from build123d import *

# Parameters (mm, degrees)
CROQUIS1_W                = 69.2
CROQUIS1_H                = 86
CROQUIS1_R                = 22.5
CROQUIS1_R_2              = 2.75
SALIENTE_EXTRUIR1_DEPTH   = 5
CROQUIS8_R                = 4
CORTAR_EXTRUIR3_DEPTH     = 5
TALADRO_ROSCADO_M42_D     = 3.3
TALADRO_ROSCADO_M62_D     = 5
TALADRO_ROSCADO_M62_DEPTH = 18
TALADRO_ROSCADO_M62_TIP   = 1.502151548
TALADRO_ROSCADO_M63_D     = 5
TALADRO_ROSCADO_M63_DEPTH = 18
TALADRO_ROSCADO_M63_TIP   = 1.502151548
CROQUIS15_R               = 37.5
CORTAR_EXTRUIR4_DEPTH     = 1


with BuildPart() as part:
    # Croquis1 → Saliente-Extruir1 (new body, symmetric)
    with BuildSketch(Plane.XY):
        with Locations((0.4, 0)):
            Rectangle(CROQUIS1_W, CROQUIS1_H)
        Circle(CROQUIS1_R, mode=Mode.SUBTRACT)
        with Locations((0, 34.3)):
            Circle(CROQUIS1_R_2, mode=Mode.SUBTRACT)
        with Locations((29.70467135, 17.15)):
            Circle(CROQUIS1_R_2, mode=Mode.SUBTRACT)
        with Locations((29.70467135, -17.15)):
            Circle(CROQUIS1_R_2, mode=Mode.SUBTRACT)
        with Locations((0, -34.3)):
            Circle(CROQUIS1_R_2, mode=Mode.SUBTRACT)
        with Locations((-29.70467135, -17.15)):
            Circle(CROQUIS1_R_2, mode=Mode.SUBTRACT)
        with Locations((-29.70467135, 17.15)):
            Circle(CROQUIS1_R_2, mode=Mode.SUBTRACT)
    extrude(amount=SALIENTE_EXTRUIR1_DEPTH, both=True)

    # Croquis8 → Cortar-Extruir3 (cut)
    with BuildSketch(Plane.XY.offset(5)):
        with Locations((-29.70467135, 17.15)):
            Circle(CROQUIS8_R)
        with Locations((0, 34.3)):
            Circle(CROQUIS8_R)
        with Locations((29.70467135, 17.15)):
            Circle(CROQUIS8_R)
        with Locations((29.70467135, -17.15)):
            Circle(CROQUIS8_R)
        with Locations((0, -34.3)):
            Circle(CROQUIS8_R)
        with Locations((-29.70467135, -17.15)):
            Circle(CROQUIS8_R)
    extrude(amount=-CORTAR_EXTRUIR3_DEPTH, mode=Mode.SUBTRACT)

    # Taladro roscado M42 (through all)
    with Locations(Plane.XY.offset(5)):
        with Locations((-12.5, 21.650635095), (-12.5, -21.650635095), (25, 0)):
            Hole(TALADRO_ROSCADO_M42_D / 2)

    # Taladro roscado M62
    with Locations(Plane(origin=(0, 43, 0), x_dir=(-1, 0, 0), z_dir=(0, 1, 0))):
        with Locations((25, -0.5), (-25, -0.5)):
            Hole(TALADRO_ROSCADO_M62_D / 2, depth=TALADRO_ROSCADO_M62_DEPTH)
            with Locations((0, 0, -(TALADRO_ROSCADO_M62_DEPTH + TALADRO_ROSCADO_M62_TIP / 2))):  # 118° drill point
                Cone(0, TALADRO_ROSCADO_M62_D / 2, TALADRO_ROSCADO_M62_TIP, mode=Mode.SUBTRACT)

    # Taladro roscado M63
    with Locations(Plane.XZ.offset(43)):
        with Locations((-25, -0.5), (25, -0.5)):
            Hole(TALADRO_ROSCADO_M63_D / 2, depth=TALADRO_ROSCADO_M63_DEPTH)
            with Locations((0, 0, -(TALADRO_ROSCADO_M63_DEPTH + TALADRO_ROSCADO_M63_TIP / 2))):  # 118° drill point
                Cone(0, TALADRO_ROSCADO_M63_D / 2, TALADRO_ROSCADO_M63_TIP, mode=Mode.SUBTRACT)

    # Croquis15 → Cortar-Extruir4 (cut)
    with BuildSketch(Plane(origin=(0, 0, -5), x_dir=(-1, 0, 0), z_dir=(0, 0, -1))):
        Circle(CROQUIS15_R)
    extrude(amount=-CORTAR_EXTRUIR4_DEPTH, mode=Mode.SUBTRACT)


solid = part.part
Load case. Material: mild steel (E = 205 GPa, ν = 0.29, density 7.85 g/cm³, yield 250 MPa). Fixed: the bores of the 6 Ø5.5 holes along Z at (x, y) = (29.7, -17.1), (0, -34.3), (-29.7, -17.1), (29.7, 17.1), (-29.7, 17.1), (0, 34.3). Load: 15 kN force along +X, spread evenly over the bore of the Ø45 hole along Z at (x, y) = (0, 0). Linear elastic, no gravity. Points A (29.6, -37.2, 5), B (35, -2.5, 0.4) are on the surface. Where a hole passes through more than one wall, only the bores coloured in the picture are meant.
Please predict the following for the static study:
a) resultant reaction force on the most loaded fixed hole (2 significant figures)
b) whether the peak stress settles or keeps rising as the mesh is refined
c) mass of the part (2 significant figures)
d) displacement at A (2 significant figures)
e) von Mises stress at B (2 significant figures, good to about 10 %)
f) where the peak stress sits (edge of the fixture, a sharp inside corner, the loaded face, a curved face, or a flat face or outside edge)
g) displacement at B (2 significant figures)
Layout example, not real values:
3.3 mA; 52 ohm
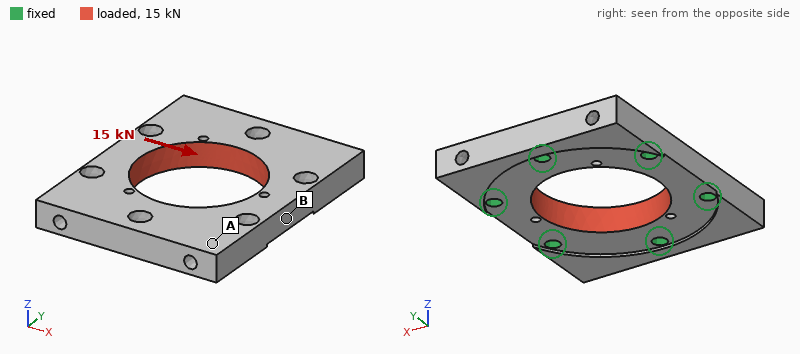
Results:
2.7 kN; keeps rising; 290 g; 2.4 µm; 21 MPa; edge of the fixture; 3.1 µm
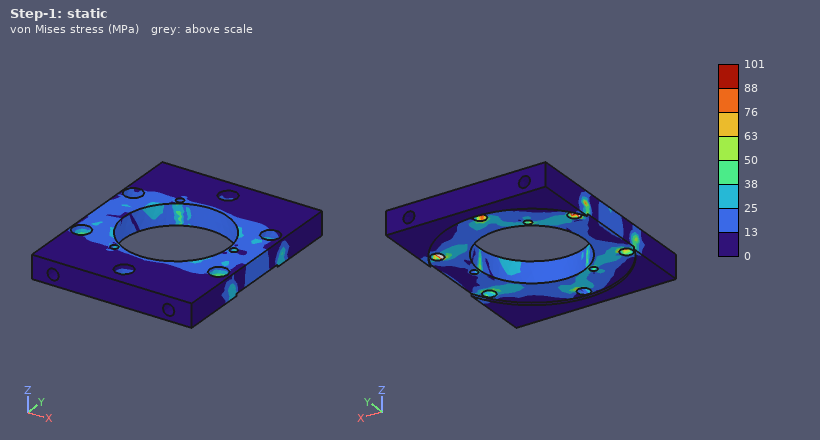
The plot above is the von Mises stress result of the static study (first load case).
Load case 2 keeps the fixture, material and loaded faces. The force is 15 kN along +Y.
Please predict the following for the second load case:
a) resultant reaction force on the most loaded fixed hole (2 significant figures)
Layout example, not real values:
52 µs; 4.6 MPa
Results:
2.9 kN
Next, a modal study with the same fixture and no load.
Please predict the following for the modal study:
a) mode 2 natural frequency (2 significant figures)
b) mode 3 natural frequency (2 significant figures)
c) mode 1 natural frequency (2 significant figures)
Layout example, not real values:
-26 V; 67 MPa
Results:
11 kHz; 11 kHz; 11 kHz
